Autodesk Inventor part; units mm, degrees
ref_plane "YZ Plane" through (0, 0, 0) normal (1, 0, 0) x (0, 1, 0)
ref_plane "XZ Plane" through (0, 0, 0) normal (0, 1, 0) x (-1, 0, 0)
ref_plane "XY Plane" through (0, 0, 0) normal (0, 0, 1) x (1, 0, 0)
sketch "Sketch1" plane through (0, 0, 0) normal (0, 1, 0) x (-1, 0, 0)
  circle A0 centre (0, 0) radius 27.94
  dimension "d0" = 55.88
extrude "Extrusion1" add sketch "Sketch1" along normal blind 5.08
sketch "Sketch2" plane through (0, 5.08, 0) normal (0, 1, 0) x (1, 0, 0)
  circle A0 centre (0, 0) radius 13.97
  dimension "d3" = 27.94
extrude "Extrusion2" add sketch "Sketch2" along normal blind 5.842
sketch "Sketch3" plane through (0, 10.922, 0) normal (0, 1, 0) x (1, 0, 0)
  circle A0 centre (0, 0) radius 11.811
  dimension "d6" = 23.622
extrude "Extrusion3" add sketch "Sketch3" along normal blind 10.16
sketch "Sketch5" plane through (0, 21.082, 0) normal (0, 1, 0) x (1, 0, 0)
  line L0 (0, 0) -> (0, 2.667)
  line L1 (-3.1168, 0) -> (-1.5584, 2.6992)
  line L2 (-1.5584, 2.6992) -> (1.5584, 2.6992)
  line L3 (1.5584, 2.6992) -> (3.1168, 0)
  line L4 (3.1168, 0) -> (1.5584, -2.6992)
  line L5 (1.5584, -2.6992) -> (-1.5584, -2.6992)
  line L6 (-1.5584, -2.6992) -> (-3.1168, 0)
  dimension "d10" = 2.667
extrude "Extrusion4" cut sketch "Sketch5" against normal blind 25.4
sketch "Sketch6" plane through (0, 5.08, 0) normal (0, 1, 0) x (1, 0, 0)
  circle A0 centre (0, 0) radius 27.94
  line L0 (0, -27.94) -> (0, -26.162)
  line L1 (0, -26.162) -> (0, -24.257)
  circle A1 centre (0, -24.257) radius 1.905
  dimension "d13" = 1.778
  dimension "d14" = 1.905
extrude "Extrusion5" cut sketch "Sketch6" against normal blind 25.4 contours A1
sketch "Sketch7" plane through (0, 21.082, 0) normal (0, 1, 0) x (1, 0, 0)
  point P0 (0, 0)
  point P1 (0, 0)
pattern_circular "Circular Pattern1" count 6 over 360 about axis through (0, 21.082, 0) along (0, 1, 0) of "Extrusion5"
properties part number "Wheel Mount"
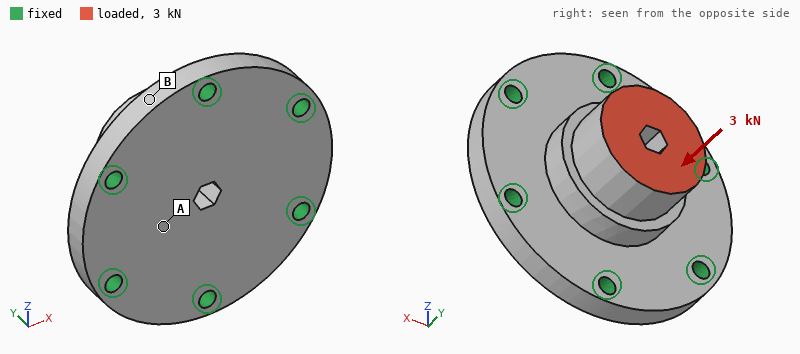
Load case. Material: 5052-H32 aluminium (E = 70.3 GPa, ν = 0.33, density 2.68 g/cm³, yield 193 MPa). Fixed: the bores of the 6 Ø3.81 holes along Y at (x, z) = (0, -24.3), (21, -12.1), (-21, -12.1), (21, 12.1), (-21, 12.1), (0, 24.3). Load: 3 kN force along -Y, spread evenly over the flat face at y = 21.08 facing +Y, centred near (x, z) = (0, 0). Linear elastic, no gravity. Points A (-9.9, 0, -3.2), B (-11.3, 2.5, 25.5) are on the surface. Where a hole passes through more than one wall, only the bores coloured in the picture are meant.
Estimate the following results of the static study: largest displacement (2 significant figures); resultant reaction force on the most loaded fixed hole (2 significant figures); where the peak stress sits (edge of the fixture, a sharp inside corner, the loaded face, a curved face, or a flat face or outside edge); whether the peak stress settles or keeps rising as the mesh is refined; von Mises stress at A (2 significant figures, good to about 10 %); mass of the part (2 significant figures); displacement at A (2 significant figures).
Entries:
12 µm
540 N
edge of the fixture
keeps rising
15 MPa
53 g
11 µm
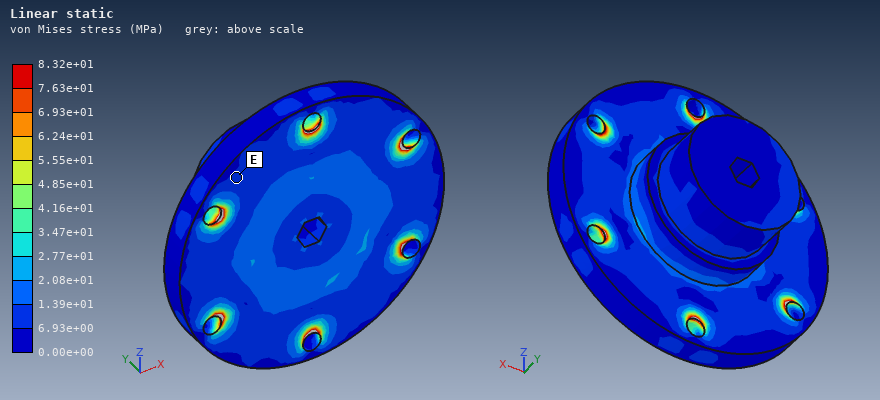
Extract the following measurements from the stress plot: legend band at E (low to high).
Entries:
6.93e+00 to 1.39e+01 MPa
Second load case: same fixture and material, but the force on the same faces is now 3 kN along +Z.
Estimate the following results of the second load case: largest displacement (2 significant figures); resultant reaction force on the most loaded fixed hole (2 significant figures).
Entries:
30 µm
1.2 kN
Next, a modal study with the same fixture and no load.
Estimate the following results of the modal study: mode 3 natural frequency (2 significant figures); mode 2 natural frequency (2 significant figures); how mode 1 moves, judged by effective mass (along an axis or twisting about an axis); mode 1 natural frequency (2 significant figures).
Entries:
17 kHz
17 kHz
along Y
15 kHz
